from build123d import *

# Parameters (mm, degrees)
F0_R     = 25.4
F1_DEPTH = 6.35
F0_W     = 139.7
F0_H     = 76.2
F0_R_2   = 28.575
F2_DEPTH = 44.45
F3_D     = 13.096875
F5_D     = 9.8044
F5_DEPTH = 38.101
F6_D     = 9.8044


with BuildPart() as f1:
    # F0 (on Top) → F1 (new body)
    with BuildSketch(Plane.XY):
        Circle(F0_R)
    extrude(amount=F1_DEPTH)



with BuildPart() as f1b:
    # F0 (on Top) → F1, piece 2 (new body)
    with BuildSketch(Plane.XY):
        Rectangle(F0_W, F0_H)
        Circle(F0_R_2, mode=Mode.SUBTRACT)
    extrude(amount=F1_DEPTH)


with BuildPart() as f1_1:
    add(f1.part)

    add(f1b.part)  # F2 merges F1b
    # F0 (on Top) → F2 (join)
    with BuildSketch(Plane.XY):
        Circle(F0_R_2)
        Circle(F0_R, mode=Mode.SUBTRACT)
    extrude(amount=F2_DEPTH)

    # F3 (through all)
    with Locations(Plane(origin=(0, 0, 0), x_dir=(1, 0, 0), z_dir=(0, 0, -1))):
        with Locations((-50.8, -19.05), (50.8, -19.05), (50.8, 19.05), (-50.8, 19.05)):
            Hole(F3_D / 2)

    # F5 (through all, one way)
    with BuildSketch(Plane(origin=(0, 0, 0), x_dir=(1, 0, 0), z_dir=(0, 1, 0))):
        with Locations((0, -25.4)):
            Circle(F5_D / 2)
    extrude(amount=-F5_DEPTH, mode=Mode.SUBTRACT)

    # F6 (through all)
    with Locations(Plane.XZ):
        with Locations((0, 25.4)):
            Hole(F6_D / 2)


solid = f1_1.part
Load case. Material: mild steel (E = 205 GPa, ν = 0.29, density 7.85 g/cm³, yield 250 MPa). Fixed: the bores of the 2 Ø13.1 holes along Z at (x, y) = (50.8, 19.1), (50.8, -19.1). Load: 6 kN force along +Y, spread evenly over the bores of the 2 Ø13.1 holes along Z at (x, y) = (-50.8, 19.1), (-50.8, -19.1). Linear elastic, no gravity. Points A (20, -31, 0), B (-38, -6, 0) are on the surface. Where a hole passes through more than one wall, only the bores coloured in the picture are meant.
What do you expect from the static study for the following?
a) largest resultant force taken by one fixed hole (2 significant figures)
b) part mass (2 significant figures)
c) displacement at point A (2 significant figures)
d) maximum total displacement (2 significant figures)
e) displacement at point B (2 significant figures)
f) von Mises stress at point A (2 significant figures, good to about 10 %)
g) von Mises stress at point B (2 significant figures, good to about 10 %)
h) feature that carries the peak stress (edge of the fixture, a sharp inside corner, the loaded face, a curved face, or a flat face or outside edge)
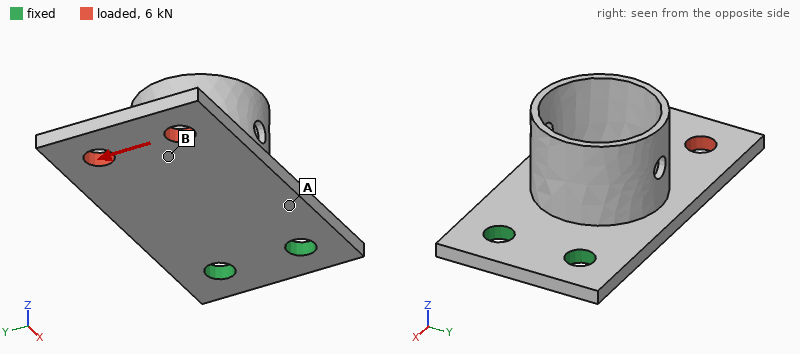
13 kN
660 g
18 µm
87 µm
56 µm
54 MPa
27 MPa
edge of the fixture
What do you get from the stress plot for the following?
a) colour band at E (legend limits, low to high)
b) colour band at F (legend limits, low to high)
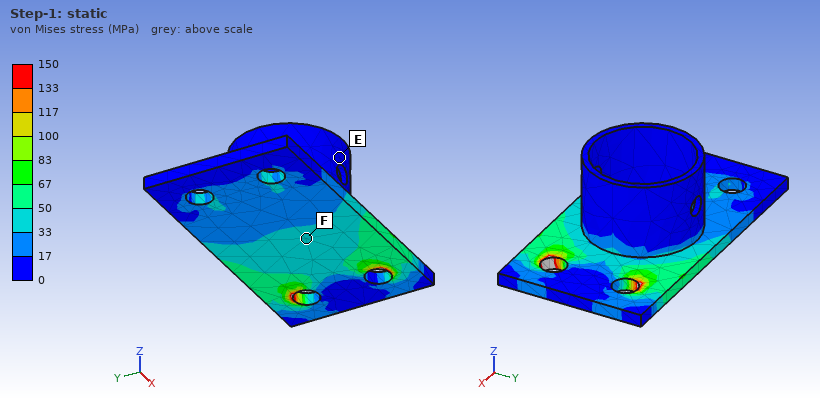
0 to 17 MPa
33 to 50 MPa
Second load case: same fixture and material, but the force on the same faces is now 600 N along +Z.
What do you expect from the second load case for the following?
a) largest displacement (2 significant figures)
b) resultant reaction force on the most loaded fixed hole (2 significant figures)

0.52 mm
310 N
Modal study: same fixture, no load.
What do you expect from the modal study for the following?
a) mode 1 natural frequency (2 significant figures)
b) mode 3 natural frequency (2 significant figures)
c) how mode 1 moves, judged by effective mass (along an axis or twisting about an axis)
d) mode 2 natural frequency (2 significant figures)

420 Hz
2500 Hz
along Z
1500 Hz
